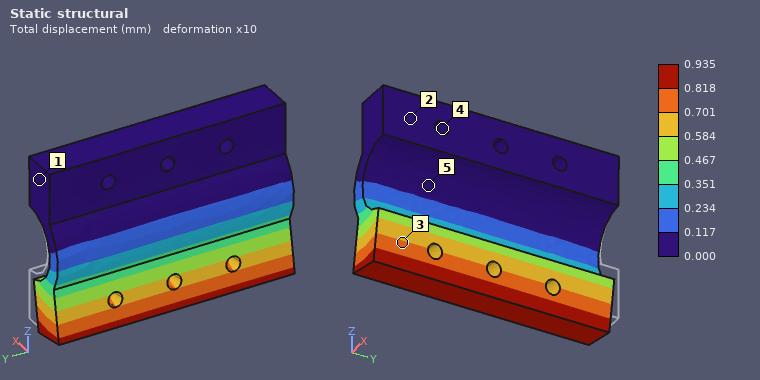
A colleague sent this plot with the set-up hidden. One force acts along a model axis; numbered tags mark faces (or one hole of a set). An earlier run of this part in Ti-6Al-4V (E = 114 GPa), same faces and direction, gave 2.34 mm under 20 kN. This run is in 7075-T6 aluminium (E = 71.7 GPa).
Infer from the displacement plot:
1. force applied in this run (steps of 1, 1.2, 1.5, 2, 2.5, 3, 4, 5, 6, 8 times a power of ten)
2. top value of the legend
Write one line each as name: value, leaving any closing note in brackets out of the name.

force applied in this run: 5 kN
top value of the legend: 0.935 mm
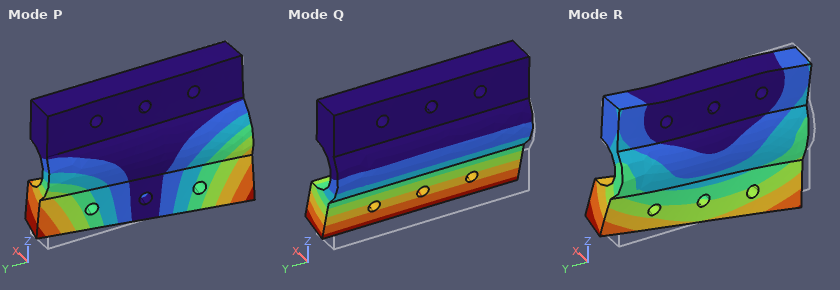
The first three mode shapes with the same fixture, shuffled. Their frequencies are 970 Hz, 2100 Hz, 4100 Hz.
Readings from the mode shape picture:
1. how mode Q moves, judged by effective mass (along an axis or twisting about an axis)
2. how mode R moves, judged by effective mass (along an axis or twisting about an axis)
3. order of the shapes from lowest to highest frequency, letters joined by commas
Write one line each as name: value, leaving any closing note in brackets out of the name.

how mode Q moves, judged by effective mass: along X
how mode R moves, judged by effective mass: along Y
order of the shapes from lowest to highest frequency, letters joined by commas: Q, P, R
